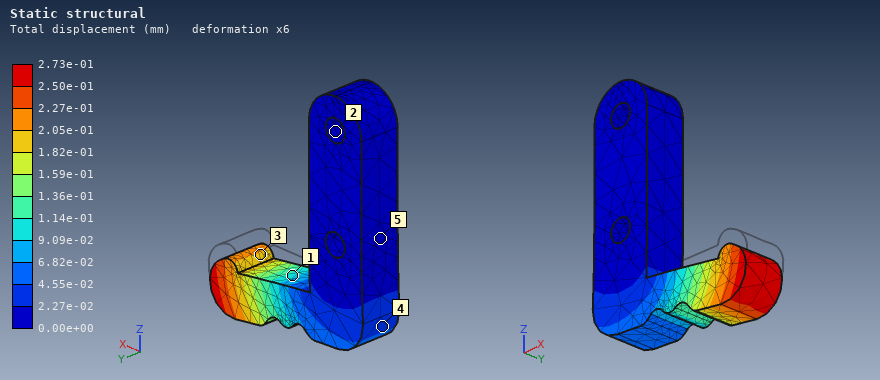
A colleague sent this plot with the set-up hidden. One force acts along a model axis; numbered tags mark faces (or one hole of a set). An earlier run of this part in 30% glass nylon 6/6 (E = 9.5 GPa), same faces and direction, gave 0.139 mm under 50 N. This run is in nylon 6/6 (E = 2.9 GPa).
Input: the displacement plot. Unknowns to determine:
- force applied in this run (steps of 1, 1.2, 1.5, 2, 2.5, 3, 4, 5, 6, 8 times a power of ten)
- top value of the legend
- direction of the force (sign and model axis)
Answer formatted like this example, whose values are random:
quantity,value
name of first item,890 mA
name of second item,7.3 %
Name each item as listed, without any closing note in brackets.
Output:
quantity,value
force applied in this run,30 N
top value of the legend,2.73e-01 mm
direction of the force,-Z
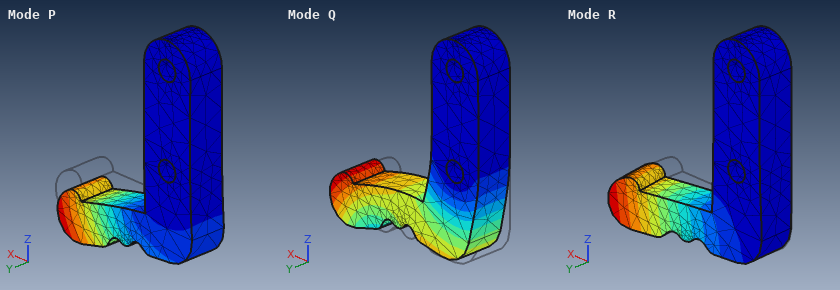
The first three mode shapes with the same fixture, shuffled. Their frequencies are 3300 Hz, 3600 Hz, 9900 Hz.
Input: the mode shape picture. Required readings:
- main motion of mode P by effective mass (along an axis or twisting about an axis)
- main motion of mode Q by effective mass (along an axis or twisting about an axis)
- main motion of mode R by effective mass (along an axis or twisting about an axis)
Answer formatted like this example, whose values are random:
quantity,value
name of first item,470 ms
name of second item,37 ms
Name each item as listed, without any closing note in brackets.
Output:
quantity,value
main motion of mode P by effective mass,along Z
main motion of mode Q by effective mass,along X
main motion of mode R by effective mass,along Y
